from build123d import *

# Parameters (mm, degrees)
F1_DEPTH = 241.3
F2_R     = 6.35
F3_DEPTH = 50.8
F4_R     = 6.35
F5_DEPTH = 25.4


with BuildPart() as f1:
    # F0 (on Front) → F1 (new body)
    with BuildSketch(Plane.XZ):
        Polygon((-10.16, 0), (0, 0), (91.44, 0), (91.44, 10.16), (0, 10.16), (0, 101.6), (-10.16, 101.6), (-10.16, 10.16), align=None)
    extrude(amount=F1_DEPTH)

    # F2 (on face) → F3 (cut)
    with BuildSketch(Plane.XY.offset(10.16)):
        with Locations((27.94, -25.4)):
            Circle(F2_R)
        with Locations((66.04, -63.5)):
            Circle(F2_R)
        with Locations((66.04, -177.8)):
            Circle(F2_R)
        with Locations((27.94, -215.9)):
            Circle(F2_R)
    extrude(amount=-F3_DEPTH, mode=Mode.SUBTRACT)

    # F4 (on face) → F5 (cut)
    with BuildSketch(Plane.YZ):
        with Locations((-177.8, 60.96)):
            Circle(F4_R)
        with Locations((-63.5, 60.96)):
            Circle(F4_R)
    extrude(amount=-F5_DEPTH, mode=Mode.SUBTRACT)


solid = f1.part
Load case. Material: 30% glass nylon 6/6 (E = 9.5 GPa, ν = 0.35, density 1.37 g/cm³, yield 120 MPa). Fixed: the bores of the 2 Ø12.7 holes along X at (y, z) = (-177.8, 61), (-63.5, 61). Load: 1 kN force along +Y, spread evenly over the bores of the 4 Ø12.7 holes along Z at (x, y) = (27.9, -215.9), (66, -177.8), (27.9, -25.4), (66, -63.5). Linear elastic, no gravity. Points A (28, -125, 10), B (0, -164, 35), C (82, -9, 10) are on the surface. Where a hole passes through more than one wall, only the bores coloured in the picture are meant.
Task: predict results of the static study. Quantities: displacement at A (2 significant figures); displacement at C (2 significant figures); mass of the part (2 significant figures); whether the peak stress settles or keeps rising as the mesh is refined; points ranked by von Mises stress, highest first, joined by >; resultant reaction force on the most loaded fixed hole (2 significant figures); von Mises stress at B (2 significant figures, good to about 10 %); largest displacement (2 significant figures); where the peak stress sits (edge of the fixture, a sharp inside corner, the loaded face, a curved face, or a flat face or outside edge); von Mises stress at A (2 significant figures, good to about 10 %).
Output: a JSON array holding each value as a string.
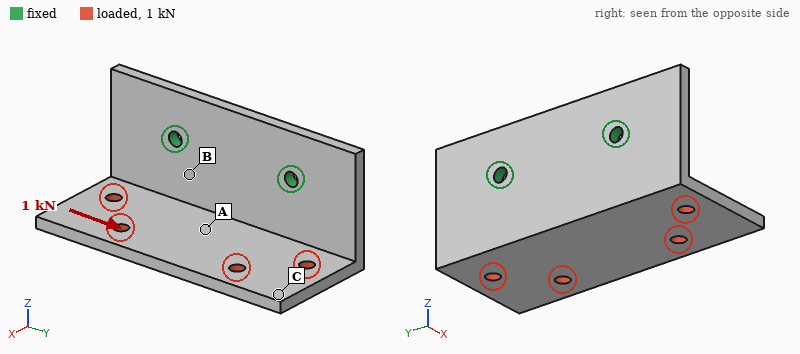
["0.11 mm", "0.46 mm", "640 g", "keeps rising", "B > A > C", "770 N", "5.3 MPa", "0.51 mm", "edge of the fixture", "2.8 MPa"]
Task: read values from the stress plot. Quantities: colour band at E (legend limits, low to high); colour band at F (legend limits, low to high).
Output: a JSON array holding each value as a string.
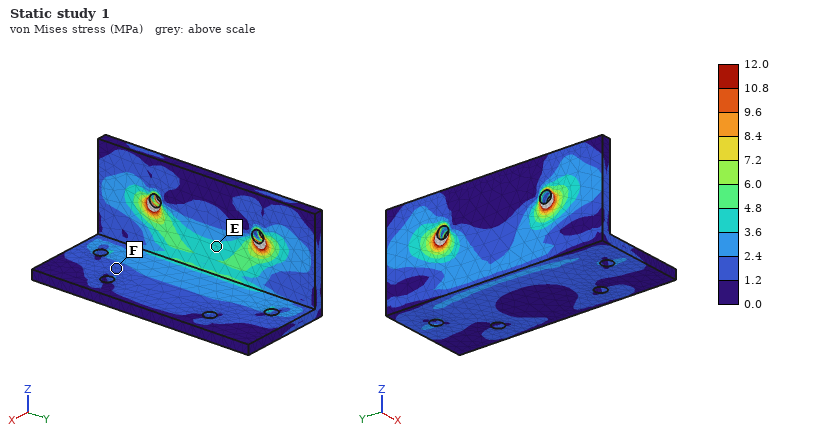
["3.6 to 4.8 MPa", "1.2 to 2.4 MPa"]
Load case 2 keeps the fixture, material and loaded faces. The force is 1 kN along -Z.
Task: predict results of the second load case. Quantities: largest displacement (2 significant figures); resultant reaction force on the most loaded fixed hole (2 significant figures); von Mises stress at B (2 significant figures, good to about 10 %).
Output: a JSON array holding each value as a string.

["2.0 mm", "500 N", "13 MPa"]
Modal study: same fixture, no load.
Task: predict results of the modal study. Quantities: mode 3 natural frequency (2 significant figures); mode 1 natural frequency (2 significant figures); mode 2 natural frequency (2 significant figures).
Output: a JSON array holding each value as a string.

["610 Hz", "230 Hz", "360 Hz"]
